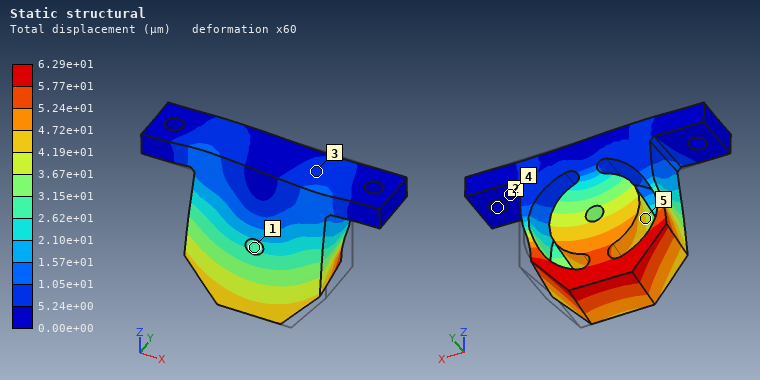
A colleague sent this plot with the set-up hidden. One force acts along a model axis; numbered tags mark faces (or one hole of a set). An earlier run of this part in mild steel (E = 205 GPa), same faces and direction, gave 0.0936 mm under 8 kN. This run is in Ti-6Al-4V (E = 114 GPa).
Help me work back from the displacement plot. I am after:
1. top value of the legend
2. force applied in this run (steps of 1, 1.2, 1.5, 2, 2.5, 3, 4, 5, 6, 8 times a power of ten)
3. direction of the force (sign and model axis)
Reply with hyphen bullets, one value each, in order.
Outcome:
- 6.29e+01 µm
- 3 kN
- -X
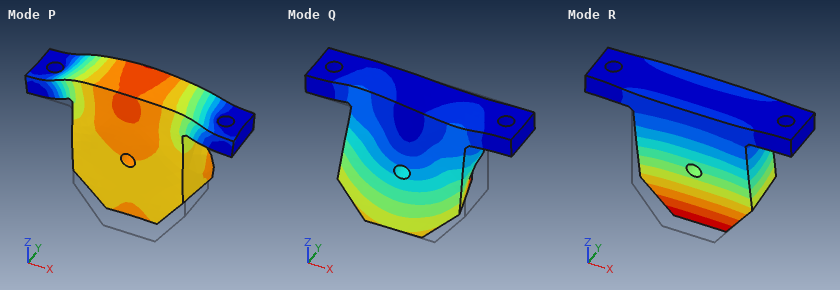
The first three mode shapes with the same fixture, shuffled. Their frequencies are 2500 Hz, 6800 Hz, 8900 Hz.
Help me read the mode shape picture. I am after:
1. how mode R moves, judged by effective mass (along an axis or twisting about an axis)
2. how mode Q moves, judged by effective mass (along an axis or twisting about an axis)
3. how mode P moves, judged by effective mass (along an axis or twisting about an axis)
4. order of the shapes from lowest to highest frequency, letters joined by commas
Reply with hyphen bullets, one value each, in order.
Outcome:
- along Y
- along X
- along Z
- R, Q, P
